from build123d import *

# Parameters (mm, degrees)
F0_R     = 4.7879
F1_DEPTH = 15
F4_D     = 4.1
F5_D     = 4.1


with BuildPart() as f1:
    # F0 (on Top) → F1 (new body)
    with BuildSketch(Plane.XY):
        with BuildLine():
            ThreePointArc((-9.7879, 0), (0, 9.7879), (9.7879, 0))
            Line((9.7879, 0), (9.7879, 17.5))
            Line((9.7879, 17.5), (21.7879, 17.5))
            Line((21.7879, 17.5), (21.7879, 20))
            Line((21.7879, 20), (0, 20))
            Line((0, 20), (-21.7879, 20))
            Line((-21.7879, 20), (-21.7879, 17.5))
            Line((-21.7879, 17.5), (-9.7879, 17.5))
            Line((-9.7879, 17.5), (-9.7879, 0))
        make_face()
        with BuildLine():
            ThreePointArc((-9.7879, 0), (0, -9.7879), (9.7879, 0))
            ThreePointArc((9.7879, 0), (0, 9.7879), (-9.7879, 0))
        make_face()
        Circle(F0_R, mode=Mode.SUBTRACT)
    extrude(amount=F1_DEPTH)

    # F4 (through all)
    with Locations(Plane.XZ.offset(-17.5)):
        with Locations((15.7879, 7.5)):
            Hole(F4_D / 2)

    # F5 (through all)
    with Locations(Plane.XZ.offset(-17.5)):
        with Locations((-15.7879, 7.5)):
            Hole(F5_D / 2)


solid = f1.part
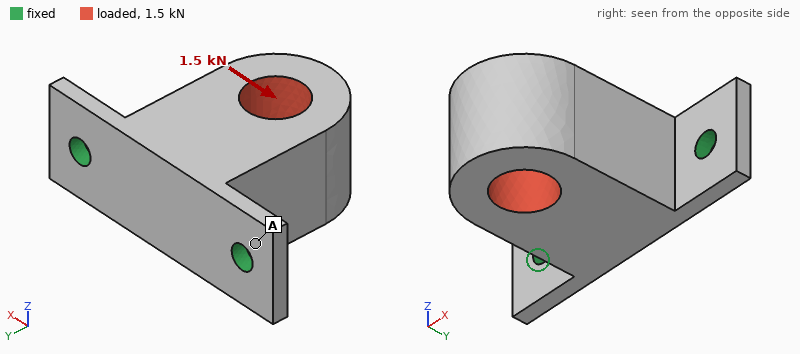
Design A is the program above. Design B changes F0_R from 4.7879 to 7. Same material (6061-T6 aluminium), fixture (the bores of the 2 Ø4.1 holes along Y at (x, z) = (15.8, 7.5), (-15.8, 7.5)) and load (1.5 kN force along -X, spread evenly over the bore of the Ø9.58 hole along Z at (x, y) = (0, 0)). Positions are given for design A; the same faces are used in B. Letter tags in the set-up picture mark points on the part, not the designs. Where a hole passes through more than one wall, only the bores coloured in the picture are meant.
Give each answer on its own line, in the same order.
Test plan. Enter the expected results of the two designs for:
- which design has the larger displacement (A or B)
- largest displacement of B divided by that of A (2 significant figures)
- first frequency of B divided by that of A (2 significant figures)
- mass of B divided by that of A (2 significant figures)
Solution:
B
1.2
1.2
0.84
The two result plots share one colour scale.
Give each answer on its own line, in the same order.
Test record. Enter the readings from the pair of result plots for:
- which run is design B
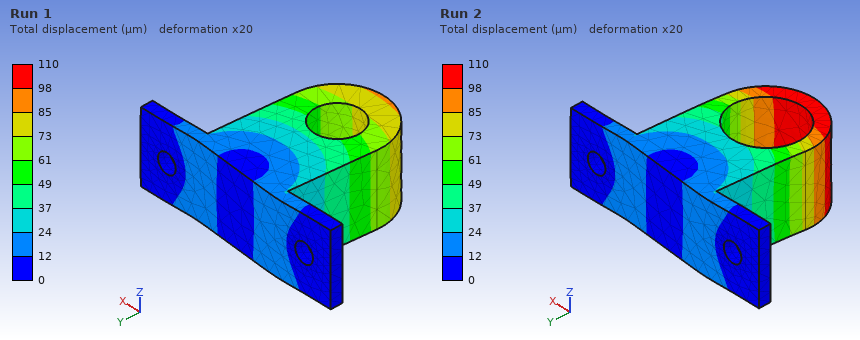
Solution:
Run 2
